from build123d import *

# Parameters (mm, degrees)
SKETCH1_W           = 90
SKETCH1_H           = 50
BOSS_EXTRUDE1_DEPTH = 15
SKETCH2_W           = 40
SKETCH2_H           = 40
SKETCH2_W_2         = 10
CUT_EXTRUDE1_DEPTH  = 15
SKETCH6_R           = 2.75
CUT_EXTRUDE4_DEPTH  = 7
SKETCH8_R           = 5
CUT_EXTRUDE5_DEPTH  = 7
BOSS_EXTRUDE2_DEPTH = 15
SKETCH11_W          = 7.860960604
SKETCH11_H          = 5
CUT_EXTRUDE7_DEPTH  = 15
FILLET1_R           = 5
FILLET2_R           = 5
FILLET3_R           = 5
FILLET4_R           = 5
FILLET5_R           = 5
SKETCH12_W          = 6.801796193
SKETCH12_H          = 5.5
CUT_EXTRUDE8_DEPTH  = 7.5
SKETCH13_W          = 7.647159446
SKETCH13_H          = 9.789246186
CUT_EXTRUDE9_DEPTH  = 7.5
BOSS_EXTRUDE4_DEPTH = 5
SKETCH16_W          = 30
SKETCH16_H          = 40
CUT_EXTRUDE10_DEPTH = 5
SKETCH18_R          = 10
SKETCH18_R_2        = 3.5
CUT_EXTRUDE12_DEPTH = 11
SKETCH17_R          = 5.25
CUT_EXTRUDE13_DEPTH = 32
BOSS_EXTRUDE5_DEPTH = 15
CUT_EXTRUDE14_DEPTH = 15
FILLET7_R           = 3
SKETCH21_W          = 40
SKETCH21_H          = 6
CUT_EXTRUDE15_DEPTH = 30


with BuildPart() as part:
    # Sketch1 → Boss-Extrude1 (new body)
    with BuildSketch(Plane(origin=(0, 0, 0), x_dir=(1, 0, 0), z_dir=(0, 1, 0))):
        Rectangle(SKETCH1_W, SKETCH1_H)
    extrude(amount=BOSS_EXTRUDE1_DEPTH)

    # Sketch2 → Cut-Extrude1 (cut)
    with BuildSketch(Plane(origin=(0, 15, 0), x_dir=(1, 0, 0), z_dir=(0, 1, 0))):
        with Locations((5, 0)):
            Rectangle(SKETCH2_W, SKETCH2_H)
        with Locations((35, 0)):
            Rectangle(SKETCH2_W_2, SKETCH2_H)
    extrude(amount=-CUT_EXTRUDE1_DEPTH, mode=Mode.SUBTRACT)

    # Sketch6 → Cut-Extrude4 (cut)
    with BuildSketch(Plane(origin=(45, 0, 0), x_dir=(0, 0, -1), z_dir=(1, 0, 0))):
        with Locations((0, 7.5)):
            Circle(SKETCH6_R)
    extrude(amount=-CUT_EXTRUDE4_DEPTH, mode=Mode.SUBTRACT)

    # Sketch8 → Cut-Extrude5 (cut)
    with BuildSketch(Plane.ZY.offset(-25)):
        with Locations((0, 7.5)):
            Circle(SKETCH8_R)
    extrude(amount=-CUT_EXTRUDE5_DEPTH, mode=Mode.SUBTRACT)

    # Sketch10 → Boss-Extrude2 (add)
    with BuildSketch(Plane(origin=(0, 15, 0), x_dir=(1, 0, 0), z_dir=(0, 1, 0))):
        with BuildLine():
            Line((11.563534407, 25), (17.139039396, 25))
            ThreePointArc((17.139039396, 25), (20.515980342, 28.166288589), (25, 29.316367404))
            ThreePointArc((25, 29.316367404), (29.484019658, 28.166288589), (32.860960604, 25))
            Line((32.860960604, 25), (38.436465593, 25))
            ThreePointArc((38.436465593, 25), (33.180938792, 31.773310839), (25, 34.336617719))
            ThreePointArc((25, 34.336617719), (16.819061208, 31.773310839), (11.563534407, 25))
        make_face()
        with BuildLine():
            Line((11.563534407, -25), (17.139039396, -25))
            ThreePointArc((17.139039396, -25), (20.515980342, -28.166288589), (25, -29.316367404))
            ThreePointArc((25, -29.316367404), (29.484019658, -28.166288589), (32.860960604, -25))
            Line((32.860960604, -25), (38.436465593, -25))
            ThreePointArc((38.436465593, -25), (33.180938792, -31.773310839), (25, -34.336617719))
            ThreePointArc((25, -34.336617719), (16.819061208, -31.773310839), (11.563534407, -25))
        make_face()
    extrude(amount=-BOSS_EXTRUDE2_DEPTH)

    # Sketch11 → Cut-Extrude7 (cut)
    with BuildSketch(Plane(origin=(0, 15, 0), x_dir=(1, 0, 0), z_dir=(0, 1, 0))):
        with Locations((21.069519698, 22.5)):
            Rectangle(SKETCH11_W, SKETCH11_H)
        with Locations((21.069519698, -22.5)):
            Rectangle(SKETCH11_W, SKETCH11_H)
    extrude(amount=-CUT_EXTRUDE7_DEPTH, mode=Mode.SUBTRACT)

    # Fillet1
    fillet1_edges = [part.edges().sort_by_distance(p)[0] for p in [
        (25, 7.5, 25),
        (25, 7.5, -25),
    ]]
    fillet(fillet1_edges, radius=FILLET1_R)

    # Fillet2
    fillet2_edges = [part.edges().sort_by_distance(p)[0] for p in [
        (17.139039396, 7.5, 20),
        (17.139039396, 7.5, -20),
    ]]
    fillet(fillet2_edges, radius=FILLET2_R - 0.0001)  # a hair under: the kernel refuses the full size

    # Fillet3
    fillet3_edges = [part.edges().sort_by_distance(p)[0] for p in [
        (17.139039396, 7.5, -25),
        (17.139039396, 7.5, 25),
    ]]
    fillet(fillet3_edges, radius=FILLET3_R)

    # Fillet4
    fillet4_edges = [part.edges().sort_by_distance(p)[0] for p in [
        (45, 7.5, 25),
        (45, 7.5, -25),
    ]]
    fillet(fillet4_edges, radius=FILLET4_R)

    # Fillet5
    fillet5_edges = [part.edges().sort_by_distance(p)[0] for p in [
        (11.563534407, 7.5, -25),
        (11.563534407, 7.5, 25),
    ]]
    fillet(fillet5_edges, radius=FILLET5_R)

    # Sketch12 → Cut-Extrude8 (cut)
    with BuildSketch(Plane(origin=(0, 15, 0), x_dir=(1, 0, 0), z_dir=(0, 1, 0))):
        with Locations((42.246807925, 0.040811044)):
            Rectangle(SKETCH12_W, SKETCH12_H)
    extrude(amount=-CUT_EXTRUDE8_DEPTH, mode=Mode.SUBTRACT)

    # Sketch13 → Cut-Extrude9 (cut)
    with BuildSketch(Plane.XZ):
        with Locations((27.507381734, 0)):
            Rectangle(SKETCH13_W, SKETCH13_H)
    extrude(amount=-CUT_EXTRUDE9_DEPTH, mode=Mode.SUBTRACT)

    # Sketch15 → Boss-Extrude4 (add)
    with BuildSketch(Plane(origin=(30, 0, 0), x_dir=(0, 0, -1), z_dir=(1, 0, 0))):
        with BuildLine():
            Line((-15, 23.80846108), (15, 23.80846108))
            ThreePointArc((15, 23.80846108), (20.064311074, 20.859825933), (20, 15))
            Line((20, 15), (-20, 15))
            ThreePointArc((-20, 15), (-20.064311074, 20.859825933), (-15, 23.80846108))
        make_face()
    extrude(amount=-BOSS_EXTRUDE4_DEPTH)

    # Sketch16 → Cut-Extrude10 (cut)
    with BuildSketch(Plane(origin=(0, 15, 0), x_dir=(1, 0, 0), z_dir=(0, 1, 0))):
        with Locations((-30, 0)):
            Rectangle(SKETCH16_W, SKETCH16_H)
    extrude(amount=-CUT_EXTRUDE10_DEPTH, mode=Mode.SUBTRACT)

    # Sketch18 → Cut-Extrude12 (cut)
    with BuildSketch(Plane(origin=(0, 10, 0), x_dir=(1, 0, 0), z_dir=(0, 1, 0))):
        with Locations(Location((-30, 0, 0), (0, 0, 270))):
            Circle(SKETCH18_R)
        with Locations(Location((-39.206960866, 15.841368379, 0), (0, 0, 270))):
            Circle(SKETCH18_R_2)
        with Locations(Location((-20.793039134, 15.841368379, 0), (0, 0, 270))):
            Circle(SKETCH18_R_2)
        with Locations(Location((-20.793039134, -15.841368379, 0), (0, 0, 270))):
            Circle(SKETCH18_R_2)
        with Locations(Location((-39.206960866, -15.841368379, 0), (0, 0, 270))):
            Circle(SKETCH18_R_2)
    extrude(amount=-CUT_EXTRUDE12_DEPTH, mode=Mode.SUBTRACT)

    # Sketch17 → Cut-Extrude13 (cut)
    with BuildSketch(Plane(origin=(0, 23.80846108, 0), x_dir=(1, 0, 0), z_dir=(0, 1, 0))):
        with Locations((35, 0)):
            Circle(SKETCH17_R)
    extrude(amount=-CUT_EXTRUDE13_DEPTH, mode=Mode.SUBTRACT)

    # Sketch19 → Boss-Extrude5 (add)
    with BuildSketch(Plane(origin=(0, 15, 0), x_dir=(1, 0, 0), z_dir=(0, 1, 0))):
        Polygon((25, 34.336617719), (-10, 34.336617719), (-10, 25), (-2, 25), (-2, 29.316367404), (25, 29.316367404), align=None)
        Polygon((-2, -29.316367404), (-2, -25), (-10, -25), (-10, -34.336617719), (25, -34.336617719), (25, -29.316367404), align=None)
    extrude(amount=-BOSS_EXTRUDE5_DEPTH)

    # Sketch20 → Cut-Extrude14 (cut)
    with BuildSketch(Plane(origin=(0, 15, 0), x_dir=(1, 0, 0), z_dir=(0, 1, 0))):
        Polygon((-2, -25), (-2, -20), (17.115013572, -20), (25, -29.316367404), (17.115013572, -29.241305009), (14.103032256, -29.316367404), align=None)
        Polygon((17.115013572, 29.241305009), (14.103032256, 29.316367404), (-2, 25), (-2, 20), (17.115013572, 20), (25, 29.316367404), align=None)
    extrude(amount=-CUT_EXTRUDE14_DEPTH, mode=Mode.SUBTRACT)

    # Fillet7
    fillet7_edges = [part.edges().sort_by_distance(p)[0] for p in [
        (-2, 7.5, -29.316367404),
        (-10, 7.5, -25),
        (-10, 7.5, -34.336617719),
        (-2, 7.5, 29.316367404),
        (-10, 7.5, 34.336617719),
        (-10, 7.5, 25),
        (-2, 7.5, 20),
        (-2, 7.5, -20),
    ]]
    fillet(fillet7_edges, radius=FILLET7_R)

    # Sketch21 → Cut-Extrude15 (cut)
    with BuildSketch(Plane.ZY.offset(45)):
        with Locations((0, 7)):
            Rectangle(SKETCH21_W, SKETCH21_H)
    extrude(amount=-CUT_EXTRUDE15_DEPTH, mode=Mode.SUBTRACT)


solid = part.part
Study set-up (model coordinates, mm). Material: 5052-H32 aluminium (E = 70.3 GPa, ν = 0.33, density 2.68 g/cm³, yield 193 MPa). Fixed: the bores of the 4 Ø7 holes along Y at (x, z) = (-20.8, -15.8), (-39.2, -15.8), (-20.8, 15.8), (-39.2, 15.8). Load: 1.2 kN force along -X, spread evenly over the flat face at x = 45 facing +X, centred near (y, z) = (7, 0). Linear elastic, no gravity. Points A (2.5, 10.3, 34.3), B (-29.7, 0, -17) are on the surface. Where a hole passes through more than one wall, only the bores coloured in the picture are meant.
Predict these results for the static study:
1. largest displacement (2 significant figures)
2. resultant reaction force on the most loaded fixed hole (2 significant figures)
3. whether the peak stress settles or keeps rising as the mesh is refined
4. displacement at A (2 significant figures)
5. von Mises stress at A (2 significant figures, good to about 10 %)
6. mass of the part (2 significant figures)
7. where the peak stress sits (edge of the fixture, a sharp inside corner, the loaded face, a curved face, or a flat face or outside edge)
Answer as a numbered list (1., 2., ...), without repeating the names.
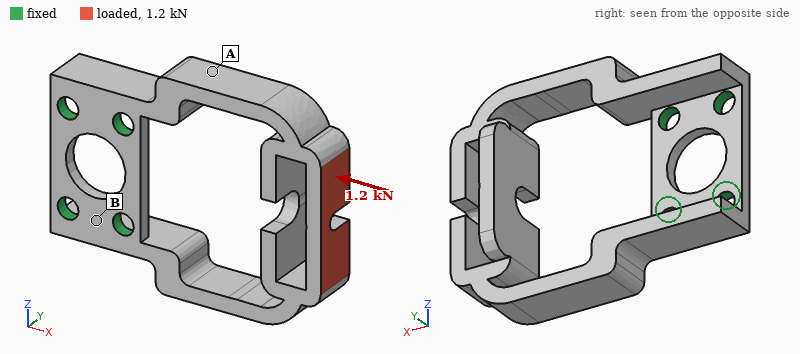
1. 0.16 mm
2. 400 N
3. keeps rising
4. 0.054 mm
5. 28 MPa
6. 73 g
7. a sharp inside corner
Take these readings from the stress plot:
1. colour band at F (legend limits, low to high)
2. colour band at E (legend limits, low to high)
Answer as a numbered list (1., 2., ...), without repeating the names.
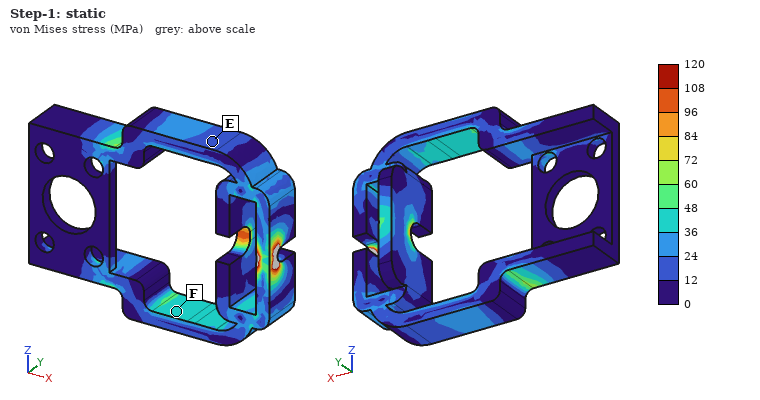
1. 36 to 48 MPa
2. 12 to 24 MPa
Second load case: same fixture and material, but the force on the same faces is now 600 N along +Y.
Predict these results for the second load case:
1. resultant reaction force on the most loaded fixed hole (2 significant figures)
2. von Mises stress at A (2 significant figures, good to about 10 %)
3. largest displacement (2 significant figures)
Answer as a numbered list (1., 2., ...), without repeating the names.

1. 1.3 kN
2. 37 MPa
3. 0.55 mm
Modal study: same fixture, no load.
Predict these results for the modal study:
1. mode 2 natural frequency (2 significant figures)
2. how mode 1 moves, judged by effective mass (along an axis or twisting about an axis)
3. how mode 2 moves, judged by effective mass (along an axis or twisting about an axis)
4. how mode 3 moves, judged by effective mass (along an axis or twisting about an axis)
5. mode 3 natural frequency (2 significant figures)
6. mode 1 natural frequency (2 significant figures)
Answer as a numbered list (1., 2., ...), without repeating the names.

1. 1200 Hz
2. along Z
3. along Y
4. twisting about X
5. 2100 Hz
6. 850 Hz
